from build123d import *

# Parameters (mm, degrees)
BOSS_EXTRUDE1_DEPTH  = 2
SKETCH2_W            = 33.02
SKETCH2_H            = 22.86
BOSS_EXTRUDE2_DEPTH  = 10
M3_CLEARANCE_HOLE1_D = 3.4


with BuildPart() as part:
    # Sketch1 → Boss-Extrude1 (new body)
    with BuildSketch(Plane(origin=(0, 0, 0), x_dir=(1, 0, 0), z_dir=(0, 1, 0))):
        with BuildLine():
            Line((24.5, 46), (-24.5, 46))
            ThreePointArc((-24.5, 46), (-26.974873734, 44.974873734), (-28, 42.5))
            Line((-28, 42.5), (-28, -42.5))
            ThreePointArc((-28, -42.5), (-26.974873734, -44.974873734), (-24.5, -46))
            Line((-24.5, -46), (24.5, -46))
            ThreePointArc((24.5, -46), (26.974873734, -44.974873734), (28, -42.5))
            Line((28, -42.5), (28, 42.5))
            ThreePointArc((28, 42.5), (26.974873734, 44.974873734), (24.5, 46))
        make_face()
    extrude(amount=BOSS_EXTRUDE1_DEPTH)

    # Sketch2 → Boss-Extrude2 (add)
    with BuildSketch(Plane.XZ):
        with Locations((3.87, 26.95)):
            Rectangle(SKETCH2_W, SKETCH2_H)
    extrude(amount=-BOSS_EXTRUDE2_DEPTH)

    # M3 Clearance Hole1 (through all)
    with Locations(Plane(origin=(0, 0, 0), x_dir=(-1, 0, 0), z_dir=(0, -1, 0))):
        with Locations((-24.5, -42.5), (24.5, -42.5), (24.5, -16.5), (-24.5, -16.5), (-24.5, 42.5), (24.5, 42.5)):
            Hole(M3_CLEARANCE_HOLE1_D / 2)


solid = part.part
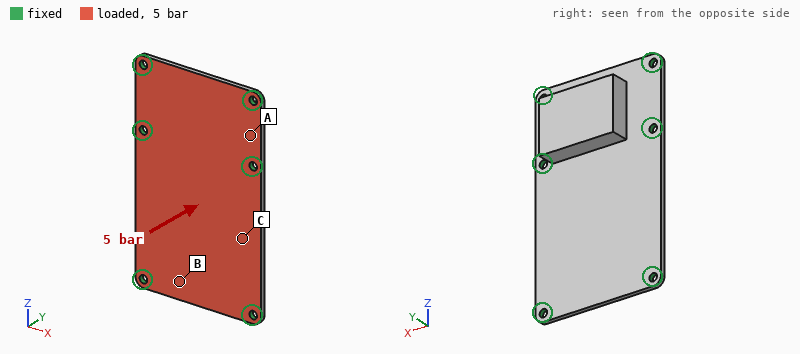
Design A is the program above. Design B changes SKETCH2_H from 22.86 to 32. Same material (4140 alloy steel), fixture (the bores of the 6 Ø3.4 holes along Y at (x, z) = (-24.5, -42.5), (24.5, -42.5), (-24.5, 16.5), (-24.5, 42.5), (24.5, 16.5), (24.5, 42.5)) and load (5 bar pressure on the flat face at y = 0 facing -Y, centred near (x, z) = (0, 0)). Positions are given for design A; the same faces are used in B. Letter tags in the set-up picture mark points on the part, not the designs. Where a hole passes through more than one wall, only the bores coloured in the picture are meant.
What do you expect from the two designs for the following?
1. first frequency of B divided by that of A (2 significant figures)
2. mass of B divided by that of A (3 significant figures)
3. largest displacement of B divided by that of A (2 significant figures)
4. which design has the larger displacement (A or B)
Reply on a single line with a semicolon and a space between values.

1.1; 1.15; 0.85; A
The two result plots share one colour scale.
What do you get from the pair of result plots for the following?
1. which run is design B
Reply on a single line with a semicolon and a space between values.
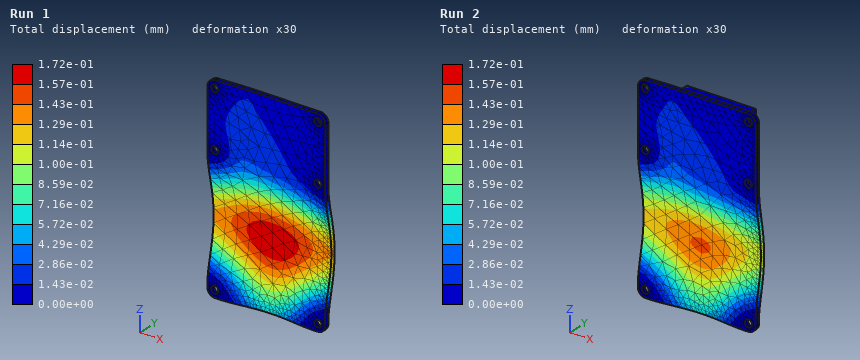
Run 2
